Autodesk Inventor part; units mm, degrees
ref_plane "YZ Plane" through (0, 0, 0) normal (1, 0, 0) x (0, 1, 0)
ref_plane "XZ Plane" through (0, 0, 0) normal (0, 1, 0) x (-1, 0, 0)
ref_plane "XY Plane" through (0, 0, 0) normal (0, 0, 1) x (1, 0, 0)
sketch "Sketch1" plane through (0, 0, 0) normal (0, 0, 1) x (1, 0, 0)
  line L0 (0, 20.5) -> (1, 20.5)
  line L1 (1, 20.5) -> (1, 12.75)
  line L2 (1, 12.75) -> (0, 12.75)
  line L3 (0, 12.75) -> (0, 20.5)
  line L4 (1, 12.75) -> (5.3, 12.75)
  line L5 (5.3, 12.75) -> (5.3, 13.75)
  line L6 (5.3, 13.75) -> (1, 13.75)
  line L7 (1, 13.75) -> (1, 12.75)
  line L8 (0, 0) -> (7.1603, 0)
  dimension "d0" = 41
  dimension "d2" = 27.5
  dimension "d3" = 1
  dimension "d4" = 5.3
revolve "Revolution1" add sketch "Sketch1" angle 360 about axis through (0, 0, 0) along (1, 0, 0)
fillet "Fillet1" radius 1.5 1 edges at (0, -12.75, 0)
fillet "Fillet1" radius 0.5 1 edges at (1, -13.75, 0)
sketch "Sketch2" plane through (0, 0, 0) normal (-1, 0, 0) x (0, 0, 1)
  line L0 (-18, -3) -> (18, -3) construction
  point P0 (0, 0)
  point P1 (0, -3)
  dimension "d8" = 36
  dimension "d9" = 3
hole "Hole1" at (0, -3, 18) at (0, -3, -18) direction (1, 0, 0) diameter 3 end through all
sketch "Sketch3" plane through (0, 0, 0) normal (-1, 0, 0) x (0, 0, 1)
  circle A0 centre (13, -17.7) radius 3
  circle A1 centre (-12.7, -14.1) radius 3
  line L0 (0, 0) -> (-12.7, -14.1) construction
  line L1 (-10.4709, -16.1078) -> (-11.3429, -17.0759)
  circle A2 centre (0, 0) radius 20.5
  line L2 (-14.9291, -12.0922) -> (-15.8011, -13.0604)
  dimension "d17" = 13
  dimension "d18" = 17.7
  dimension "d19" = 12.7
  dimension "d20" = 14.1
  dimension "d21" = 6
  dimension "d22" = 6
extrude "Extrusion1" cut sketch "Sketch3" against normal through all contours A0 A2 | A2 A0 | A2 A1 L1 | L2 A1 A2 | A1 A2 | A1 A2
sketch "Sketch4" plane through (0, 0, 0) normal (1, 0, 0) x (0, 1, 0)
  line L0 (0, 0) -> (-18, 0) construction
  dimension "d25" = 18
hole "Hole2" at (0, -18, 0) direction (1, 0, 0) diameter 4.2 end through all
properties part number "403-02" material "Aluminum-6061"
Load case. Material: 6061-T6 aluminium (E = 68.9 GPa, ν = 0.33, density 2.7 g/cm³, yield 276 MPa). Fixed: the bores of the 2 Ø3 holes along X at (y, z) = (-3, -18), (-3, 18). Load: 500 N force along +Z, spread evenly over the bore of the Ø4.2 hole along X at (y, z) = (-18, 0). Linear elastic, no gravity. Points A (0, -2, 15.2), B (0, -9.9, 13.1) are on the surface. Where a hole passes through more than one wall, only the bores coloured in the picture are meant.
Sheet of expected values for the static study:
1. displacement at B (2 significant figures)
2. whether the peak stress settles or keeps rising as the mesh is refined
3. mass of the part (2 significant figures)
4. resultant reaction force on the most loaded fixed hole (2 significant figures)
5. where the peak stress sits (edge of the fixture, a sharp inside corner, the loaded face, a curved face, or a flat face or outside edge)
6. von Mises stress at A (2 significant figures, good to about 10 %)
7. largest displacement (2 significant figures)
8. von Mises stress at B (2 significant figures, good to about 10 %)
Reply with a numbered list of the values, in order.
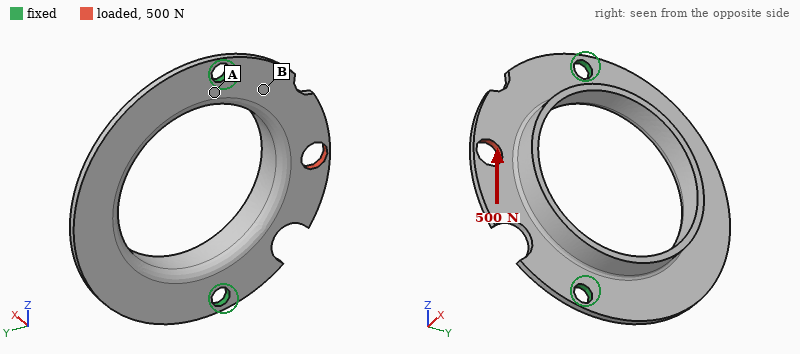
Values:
1. 17 µm
2. keeps rising
3. 2.9 g
4. 320 N
5. a sharp inside corner
6. 20 MPa
7. 35 µm
8. 53 MPa
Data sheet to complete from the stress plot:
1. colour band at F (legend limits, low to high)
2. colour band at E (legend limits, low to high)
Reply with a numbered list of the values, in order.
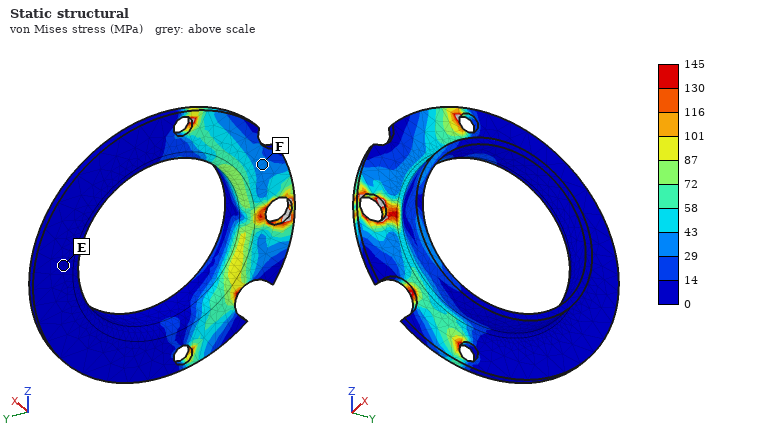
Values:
1. 29 to 43 MPa
2. 0 to 14 MPa
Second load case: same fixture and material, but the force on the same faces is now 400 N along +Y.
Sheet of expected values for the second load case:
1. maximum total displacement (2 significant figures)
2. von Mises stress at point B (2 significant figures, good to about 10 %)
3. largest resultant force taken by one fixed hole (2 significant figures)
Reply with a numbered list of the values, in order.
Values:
1. 58 µm
2. 40 MPa
3. 270 N
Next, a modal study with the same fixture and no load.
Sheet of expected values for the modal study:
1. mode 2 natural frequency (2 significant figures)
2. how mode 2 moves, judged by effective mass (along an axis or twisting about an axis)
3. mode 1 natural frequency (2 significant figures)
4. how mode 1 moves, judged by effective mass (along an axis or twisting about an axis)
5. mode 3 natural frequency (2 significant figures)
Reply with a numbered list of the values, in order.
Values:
1. 3600 Hz
2. along X
3. 1800 Hz
4. along X
5. 5300 Hz
